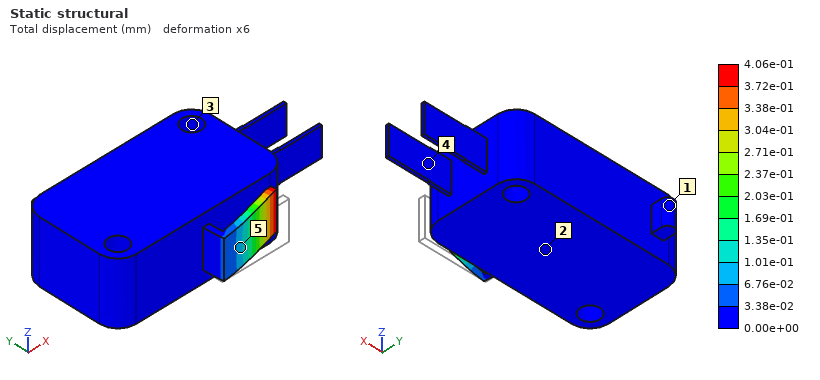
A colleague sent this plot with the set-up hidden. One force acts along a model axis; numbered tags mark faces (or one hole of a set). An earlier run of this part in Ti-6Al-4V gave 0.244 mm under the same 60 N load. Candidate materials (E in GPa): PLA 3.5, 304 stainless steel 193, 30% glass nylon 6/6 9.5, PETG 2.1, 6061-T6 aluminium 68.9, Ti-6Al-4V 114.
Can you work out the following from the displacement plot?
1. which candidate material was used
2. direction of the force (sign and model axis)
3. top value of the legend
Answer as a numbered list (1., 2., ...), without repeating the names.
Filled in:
1. 6061-T6 aluminium
2. +Y
3. 4.06e-01 mm
